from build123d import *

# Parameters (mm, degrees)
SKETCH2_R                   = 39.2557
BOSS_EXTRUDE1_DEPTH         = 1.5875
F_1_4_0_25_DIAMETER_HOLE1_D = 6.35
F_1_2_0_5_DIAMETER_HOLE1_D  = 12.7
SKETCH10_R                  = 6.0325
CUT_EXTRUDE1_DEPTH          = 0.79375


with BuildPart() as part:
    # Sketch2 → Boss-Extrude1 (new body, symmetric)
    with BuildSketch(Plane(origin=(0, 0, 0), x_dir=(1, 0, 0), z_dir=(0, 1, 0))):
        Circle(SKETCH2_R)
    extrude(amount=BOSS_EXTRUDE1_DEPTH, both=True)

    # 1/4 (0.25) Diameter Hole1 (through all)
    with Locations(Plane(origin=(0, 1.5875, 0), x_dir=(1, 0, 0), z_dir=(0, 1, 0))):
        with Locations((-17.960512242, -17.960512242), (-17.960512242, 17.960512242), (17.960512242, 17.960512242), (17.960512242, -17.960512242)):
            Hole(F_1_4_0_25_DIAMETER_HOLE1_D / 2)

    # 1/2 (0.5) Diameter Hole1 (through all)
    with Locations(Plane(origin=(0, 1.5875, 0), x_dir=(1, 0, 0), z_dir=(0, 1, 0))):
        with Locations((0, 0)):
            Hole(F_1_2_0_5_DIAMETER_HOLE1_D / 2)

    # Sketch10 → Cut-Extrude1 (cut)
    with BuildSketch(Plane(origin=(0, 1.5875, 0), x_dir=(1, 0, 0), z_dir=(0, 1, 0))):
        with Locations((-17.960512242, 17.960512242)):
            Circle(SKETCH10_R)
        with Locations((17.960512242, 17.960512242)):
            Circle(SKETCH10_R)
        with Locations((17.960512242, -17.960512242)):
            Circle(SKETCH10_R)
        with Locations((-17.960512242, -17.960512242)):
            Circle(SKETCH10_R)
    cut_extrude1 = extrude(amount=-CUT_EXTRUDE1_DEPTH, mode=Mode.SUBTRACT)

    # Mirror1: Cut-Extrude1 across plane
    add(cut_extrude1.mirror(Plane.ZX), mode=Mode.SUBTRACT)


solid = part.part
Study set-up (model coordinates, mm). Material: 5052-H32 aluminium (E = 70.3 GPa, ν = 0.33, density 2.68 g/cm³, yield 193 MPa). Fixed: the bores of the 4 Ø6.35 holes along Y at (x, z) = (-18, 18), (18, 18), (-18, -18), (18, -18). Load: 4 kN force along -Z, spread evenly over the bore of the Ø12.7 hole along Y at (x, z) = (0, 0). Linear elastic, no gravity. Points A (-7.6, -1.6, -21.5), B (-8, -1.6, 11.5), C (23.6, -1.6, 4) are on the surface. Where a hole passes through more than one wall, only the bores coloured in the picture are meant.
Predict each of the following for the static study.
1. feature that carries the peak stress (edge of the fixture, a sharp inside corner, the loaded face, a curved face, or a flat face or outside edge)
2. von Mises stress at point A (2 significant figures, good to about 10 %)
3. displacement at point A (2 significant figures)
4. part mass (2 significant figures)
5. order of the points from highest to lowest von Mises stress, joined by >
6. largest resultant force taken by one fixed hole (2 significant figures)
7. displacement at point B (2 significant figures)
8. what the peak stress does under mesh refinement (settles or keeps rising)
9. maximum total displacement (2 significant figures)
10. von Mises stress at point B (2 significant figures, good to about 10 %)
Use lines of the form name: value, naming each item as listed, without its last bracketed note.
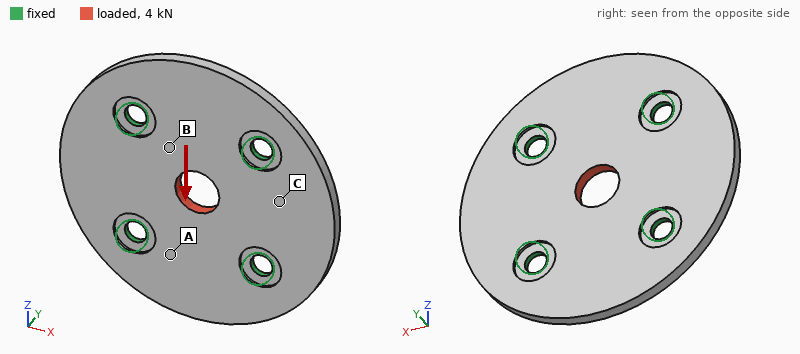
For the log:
feature that carries the peak stress: edge of the fixture
von Mises stress at point A: 12 MPa
displacement at point A: 4.2 µm
part mass: 38 g
order of the points from highest to lowest von Mises stress, joined by >: B > A > C
largest resultant force taken by one fixed hole: 1.0 kN
displacement at point B: 5.3 µm
what the peak stress does under mesh refinement: keeps rising
maximum total displacement: 9.3 µm
von Mises stress at point B: 22 MPa
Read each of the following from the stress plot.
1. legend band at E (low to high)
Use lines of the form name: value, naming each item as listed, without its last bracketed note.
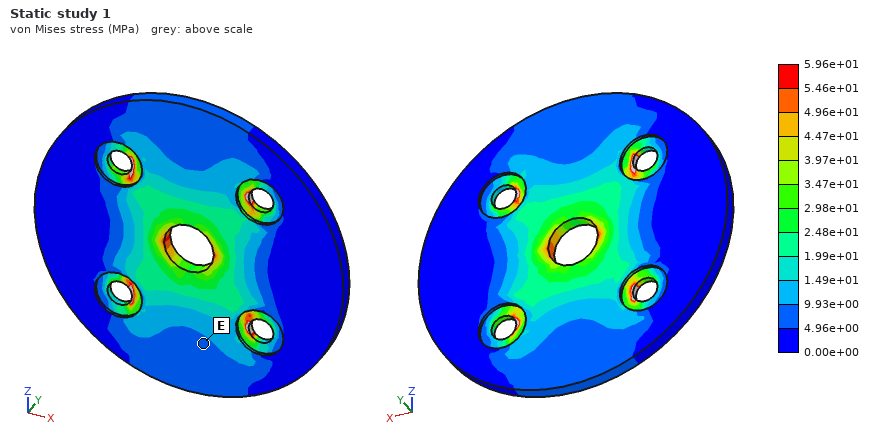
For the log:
legend band at E: 4.96e+00 to 9.93e+00 MPa
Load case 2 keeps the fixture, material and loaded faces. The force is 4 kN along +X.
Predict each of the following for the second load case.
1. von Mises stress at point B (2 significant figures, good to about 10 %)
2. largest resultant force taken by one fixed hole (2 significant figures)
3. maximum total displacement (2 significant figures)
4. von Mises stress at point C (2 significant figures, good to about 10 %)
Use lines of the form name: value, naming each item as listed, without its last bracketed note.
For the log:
von Mises stress at point B: 21 MPa
largest resultant force taken by one fixed hole: 1.0 kN
maximum total displacement: 9.3 µm
von Mises stress at point C: 9.3 MPa
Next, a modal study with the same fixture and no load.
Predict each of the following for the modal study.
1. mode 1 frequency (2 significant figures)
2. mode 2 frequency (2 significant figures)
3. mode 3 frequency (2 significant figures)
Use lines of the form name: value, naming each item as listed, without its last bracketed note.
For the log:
mode 1 frequency: 4500 Hz
mode 2 frequency: 5000 Hz
mode 3 frequency: 5000 Hz
